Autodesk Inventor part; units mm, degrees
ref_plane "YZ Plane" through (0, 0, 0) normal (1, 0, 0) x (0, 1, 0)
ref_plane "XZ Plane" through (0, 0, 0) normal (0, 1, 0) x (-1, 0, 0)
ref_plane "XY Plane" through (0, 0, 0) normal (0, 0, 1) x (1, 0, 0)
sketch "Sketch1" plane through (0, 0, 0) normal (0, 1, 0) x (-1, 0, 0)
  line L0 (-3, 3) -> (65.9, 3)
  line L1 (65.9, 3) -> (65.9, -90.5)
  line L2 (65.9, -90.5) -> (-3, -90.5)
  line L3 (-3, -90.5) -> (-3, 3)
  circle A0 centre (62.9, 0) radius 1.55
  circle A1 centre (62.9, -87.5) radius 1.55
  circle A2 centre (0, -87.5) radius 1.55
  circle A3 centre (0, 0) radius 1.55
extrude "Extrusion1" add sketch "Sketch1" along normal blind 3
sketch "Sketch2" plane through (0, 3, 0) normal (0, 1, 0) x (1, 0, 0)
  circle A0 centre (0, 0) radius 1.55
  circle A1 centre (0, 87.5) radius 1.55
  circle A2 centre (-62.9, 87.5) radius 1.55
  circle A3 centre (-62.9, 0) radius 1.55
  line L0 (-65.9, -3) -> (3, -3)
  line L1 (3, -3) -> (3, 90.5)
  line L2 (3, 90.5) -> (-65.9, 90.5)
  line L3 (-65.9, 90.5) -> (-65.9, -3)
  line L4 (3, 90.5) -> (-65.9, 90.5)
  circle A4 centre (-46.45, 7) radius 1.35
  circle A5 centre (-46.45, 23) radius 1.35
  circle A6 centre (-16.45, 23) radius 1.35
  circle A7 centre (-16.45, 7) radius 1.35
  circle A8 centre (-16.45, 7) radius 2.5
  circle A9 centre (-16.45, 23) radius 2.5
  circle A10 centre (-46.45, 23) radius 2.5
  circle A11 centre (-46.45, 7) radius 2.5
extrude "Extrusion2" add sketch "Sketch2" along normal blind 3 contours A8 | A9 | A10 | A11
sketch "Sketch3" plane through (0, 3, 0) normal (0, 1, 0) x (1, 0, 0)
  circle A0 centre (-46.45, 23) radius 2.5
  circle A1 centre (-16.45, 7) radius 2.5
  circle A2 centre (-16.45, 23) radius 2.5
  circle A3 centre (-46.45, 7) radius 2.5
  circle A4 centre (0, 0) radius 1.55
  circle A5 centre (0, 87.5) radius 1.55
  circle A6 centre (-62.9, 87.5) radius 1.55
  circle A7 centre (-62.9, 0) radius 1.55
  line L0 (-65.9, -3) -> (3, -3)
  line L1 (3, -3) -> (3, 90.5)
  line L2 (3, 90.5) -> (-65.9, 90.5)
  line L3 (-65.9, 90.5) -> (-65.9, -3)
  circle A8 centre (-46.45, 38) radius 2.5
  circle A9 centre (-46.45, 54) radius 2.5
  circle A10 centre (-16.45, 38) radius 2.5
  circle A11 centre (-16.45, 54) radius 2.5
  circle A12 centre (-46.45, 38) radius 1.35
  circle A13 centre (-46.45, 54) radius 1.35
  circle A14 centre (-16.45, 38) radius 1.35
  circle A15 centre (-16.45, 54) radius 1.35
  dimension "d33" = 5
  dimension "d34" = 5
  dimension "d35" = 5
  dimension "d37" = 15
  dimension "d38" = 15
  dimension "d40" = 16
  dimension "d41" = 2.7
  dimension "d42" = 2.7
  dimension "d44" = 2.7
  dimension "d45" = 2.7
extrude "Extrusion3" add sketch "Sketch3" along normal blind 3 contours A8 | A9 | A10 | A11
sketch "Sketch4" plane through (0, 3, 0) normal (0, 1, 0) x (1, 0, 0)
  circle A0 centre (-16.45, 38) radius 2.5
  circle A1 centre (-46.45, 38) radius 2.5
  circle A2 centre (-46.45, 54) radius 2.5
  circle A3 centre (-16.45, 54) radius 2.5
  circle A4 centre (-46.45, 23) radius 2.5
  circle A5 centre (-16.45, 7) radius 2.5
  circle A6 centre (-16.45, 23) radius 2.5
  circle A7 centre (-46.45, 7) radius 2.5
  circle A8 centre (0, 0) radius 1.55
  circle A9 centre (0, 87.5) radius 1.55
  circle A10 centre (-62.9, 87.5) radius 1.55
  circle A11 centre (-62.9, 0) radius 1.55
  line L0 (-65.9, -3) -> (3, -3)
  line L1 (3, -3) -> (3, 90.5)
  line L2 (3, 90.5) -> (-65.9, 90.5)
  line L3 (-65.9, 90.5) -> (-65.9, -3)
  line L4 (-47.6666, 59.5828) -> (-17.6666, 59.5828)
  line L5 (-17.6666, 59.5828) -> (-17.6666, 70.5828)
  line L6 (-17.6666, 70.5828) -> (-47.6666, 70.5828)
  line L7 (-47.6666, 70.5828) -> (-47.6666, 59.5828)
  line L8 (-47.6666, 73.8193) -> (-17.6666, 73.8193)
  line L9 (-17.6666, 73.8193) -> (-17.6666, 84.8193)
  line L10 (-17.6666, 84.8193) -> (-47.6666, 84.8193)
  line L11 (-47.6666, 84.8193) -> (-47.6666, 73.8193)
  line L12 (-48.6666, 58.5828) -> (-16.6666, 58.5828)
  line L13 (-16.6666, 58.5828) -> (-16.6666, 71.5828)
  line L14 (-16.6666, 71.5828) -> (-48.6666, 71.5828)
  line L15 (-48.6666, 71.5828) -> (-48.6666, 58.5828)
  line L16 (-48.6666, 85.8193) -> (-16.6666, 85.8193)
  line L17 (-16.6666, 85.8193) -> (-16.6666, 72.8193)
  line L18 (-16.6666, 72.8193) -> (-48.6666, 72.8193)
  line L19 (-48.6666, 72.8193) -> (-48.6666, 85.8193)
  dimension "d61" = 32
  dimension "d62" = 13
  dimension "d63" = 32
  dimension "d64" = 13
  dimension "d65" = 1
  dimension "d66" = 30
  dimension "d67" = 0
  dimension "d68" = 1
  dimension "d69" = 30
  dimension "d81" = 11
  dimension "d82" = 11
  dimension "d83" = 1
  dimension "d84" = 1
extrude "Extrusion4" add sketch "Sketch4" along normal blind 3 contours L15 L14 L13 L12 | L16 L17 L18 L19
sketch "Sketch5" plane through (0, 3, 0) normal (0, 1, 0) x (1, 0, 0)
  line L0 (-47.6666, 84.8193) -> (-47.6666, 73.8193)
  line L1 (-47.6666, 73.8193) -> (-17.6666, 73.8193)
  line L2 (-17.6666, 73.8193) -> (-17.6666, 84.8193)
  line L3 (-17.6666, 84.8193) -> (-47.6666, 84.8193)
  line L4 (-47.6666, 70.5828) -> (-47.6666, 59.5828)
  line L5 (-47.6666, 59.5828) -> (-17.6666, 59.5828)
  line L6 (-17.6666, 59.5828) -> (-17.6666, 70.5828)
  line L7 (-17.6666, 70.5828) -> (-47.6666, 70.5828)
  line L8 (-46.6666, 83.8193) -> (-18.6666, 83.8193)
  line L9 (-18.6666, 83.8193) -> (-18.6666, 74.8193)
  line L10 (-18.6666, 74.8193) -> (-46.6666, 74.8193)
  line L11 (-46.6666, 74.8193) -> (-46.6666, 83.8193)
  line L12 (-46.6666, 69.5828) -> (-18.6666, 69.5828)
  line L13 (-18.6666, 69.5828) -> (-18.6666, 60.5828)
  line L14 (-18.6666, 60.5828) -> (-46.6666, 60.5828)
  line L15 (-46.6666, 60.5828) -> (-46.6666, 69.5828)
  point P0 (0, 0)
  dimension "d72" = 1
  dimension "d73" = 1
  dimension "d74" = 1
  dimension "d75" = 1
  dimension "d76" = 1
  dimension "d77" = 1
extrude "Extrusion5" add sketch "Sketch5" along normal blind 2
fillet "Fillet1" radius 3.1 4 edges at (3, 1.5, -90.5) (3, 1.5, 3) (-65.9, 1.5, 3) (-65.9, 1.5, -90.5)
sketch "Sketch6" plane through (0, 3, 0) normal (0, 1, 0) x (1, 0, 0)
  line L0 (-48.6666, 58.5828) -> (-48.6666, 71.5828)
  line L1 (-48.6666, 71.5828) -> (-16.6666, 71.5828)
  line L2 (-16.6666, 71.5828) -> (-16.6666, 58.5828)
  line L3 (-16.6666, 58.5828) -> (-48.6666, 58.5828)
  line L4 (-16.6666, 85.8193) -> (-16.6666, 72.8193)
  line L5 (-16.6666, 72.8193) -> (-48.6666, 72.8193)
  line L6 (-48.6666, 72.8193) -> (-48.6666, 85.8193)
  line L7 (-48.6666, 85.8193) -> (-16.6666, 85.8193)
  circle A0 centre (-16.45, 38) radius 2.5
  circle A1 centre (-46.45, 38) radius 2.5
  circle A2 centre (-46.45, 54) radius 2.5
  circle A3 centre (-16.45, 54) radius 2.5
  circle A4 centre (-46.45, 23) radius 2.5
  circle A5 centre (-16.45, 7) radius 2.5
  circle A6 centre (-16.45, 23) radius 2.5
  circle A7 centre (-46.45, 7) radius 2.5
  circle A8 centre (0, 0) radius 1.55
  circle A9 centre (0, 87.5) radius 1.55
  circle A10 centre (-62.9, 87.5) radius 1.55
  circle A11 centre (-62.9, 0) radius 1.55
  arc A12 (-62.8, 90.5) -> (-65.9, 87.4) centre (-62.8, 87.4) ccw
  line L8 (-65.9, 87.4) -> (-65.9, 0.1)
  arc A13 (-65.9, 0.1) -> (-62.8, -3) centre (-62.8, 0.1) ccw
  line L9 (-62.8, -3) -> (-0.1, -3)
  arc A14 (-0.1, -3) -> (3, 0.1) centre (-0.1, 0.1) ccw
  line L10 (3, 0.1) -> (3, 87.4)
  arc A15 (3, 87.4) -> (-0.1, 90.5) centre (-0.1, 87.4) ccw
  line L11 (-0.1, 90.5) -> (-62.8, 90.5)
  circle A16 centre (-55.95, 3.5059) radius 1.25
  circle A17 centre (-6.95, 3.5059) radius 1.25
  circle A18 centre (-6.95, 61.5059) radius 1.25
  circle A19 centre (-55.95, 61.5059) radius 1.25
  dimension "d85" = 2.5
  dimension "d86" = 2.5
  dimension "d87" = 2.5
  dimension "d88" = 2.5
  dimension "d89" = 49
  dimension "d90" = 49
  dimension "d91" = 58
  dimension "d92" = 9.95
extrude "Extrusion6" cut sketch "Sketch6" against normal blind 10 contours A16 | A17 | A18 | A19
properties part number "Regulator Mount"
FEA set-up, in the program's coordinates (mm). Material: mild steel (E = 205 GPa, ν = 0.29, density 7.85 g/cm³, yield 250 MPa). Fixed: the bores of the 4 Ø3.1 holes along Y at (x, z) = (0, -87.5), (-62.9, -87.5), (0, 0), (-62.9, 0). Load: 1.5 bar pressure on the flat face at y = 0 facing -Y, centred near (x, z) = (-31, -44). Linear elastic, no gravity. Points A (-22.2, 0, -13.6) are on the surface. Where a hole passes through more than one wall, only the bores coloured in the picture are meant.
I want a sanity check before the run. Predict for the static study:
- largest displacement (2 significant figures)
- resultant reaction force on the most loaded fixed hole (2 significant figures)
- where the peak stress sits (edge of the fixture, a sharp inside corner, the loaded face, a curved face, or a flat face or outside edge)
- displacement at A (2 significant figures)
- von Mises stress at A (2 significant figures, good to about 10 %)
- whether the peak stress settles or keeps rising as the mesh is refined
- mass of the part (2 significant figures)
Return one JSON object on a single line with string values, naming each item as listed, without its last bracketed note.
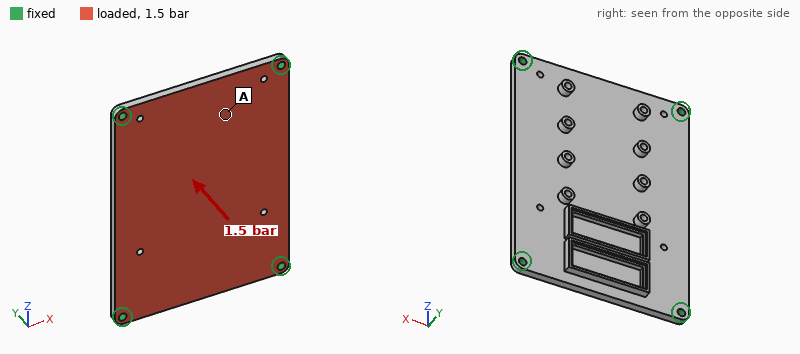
{"largest displacement": "94 µm", "resultant reaction force on the most loaded fixed hole": "250 N", "where the peak stress sits": "edge of the fixture", "displacement at A": "51 µm", "von Mises stress at A": "21 MPa", "whether the peak stress settles or keeps rising as the mesh is refined": "keeps rising", "mass of the part": "160 g"}
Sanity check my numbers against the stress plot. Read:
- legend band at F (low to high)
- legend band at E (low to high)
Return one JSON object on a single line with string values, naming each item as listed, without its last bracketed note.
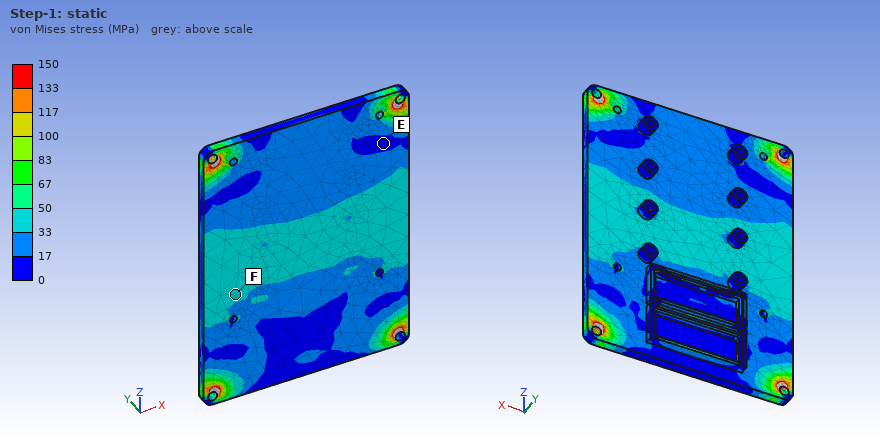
{"legend band at F": "33 to 50 MPa", "legend band at E": "0 to 17 MPa"}
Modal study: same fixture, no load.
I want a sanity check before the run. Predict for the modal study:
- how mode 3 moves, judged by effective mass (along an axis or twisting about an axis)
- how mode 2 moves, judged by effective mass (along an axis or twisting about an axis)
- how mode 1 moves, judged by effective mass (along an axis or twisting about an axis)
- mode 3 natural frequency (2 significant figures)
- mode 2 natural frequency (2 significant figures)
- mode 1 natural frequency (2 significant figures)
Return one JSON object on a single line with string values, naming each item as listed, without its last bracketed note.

{"how mode 3 moves, judged by effective mass": "twisting about X", "how mode 2 moves, judged by effective mass": "twisting about Z", "how mode 1 moves, judged by effective mass": "along Y", "mode 3 natural frequency": "3500 Hz", "mode 2 natural frequency": "2600 Hz", "mode 1 natural frequency": "1500 Hz"}
